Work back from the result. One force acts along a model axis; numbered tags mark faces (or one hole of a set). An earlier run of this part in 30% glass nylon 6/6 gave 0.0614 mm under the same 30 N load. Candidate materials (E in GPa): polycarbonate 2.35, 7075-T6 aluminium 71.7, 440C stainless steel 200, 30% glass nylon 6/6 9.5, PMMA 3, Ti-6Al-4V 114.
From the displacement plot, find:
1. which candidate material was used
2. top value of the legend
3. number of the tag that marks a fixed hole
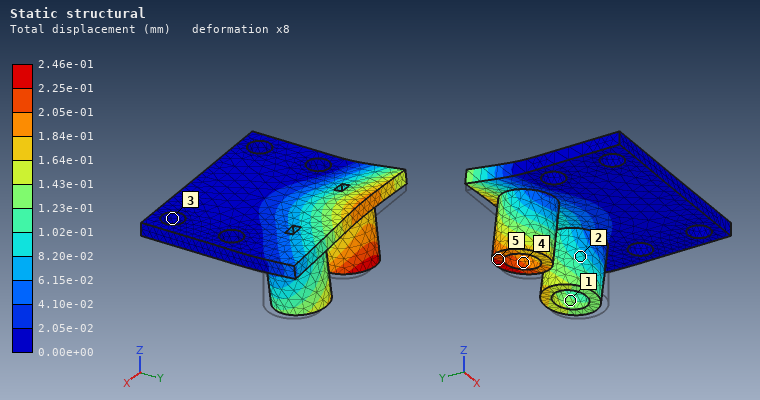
polycarbonate
2.46e-01 mm
3
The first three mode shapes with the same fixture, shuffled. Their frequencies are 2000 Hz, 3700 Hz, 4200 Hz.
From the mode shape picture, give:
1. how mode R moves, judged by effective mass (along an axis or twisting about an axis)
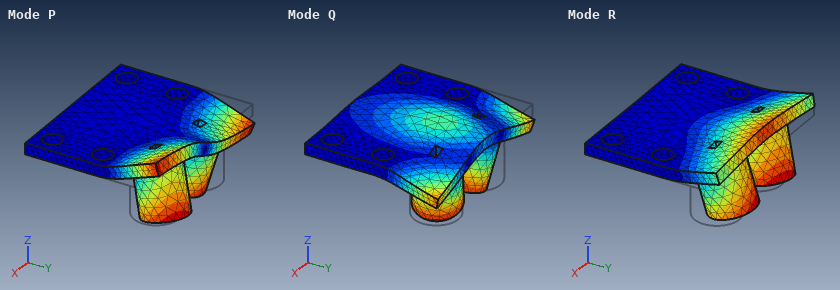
along Z
